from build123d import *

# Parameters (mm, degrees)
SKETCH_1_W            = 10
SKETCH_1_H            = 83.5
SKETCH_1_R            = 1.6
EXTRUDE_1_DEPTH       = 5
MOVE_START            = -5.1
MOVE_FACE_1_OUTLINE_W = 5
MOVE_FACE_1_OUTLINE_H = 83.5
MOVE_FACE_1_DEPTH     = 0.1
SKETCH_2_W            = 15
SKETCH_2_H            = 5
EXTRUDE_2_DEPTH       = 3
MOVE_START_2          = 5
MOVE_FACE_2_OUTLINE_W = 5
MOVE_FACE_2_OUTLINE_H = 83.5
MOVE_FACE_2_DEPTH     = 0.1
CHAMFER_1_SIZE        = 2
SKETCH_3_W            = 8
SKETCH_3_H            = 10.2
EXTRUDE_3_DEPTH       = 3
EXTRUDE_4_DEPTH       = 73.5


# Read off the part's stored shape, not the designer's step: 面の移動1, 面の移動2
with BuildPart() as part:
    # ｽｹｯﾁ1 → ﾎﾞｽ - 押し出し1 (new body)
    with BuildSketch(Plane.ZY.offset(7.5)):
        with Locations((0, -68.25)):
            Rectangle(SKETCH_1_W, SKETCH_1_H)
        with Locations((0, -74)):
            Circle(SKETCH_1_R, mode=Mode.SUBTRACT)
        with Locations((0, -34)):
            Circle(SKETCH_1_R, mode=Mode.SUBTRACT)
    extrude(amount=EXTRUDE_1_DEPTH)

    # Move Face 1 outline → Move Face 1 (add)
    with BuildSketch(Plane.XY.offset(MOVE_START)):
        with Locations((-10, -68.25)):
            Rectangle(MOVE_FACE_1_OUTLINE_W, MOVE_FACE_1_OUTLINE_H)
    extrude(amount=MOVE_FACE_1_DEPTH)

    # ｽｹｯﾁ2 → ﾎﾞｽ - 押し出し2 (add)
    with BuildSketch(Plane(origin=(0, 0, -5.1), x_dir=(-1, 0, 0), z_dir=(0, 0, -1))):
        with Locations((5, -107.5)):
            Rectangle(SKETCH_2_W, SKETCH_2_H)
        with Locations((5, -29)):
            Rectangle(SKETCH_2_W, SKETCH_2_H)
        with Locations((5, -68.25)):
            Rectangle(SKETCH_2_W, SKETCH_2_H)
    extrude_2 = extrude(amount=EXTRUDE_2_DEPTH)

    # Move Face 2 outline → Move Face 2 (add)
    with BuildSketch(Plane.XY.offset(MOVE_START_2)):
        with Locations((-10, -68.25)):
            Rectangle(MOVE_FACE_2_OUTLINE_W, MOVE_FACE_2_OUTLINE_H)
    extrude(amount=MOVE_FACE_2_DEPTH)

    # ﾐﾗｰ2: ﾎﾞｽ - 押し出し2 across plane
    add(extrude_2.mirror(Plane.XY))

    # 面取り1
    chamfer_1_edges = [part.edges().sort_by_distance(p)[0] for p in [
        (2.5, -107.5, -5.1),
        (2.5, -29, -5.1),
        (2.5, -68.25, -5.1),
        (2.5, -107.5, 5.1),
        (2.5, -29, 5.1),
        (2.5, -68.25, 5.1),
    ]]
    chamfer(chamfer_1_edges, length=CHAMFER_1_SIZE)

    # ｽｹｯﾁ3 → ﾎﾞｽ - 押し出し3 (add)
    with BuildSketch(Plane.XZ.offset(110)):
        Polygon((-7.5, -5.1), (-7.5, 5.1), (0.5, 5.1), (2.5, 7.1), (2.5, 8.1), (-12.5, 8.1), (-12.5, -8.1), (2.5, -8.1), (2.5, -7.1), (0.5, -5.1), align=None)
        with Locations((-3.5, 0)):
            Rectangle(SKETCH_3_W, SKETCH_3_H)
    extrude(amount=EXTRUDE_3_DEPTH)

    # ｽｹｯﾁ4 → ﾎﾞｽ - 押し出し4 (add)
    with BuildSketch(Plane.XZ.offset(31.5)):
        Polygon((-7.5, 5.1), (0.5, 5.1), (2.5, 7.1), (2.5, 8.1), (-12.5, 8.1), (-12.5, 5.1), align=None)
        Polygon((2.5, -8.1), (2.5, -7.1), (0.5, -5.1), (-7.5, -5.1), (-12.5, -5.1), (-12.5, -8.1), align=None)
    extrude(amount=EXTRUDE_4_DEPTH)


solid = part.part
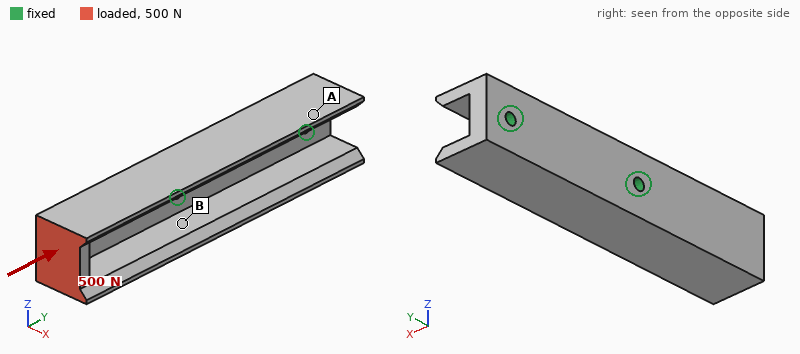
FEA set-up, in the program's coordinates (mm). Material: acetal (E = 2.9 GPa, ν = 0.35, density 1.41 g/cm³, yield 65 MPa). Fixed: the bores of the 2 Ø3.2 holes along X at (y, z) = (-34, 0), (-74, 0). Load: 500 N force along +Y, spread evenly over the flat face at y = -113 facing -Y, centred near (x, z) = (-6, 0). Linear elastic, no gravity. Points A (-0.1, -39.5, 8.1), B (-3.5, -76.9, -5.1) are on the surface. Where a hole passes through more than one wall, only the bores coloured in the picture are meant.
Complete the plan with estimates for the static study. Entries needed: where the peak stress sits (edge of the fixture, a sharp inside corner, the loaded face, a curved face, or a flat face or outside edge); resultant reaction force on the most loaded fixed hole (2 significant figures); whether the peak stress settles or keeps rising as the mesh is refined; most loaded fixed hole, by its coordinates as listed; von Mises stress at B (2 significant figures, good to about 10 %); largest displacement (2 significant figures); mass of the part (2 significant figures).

edge of the fixture
370 N
keeps rising
(-74, 0)
4.3 MPa
0.27 mm
17 g
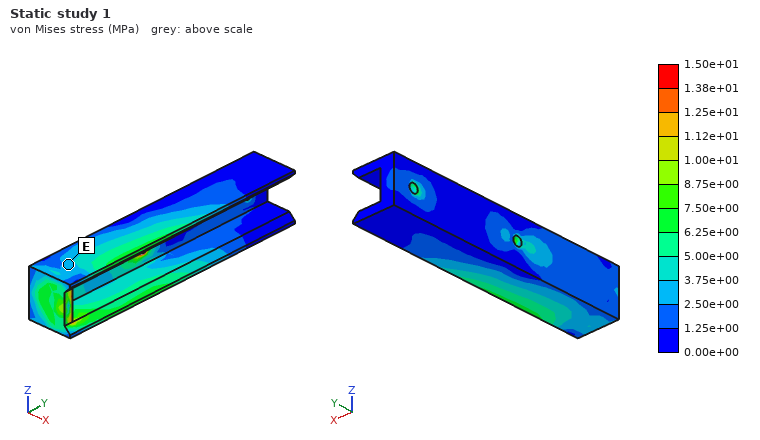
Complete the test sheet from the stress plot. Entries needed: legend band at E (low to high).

2.50e+00 to 3.75e+00 MPa
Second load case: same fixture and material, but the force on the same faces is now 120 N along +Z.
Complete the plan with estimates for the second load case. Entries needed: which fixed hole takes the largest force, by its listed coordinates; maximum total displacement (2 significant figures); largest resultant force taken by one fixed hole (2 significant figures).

(-74, 0)
0.90 mm
210 N
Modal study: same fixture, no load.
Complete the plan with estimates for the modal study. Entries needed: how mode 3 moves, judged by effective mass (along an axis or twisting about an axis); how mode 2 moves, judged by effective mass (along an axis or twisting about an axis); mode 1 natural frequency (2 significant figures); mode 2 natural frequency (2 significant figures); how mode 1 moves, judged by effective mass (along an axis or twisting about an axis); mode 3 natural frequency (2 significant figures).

twisting about Y
along X
1300 Hz
1300 Hz
along Z
2200 Hz
